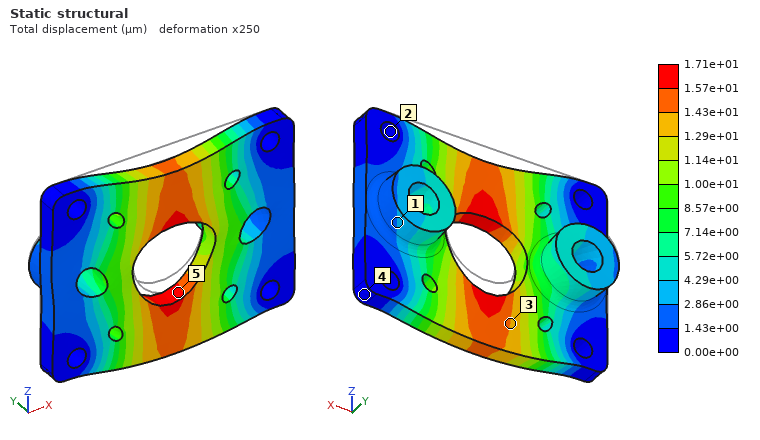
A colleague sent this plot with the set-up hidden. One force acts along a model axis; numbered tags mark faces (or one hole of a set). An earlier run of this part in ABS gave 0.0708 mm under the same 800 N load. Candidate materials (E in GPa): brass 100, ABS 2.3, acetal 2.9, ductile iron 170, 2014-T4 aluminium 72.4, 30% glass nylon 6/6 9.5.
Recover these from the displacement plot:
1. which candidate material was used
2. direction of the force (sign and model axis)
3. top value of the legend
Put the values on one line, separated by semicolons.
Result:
30% glass nylon 6/6; -Z; 1.71e+01 µm
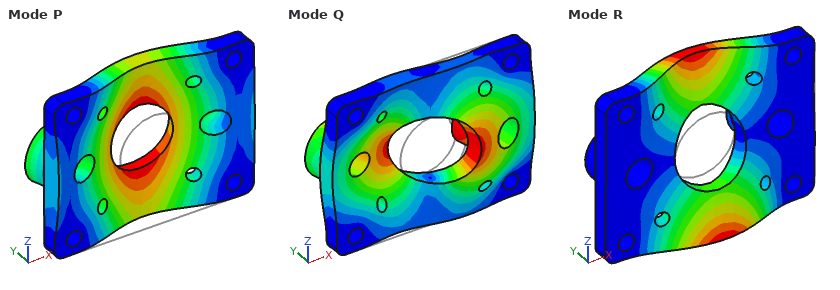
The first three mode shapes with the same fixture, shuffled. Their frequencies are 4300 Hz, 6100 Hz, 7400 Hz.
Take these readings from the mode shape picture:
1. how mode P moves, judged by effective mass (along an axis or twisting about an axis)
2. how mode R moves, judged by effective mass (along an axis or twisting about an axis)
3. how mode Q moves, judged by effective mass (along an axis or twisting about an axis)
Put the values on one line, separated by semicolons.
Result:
along Y; twisting about X; twisting about Z
